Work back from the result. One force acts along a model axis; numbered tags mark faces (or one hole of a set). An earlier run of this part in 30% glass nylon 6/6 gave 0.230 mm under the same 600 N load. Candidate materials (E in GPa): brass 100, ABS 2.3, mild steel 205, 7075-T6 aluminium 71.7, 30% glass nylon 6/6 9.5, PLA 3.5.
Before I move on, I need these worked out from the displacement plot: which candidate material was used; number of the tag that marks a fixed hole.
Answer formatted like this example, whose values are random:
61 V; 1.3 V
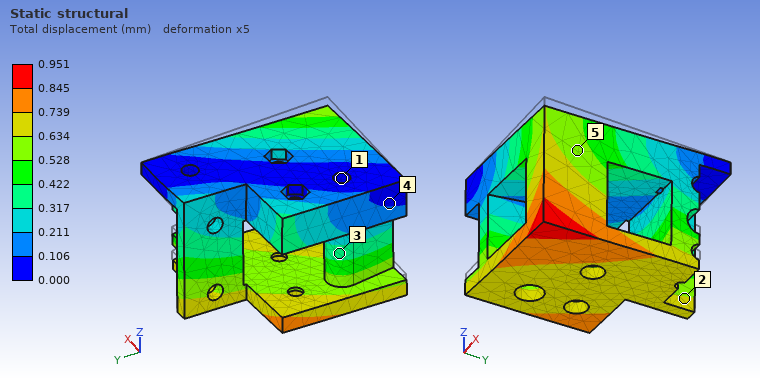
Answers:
ABS; 1
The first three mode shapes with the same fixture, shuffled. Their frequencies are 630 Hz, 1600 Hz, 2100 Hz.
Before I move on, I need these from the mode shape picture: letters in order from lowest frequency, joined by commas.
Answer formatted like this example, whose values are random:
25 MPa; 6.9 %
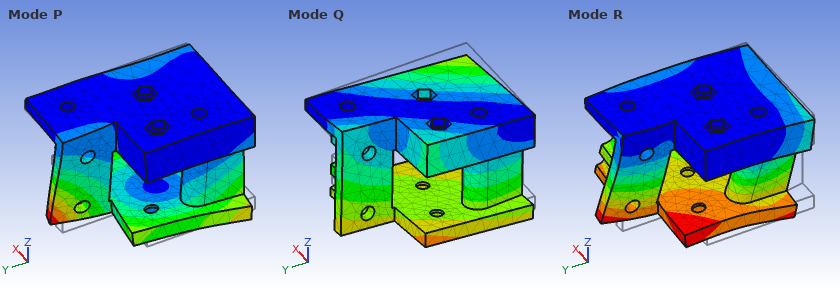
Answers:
Q, R, P
